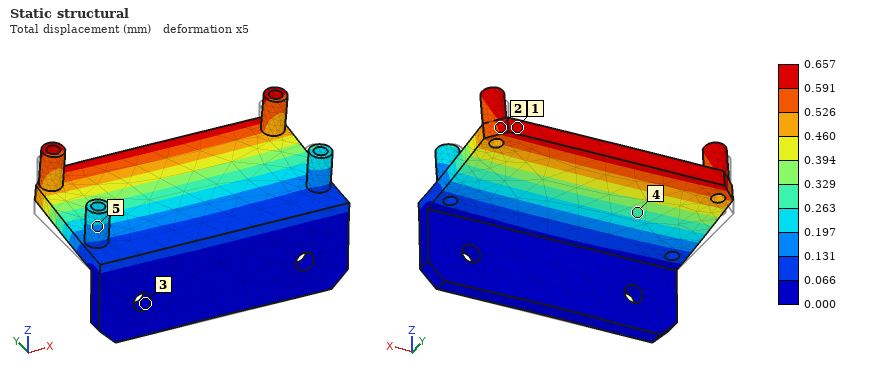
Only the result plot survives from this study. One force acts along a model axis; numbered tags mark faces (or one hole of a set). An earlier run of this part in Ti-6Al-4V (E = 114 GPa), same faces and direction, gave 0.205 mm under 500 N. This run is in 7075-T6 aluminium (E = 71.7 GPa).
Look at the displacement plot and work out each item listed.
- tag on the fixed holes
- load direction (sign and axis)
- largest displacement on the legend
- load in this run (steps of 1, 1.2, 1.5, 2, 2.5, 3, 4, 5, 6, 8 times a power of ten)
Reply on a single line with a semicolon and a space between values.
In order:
3; +Z; 0.657 mm; 1 kN
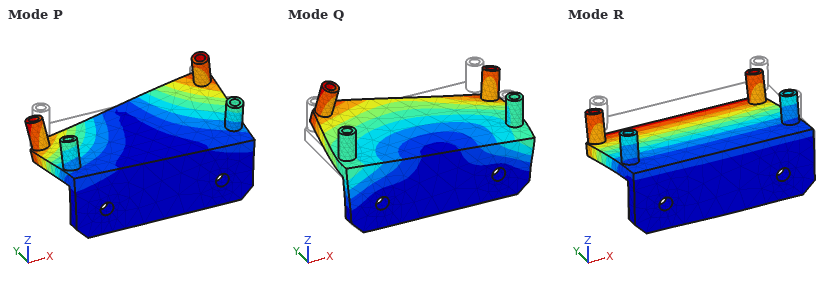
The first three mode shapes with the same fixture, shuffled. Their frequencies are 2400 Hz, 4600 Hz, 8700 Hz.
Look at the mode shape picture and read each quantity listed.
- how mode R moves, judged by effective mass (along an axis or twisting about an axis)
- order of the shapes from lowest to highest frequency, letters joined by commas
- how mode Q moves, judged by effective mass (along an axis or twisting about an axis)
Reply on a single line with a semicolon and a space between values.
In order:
along Z; R, P, Q; along X
